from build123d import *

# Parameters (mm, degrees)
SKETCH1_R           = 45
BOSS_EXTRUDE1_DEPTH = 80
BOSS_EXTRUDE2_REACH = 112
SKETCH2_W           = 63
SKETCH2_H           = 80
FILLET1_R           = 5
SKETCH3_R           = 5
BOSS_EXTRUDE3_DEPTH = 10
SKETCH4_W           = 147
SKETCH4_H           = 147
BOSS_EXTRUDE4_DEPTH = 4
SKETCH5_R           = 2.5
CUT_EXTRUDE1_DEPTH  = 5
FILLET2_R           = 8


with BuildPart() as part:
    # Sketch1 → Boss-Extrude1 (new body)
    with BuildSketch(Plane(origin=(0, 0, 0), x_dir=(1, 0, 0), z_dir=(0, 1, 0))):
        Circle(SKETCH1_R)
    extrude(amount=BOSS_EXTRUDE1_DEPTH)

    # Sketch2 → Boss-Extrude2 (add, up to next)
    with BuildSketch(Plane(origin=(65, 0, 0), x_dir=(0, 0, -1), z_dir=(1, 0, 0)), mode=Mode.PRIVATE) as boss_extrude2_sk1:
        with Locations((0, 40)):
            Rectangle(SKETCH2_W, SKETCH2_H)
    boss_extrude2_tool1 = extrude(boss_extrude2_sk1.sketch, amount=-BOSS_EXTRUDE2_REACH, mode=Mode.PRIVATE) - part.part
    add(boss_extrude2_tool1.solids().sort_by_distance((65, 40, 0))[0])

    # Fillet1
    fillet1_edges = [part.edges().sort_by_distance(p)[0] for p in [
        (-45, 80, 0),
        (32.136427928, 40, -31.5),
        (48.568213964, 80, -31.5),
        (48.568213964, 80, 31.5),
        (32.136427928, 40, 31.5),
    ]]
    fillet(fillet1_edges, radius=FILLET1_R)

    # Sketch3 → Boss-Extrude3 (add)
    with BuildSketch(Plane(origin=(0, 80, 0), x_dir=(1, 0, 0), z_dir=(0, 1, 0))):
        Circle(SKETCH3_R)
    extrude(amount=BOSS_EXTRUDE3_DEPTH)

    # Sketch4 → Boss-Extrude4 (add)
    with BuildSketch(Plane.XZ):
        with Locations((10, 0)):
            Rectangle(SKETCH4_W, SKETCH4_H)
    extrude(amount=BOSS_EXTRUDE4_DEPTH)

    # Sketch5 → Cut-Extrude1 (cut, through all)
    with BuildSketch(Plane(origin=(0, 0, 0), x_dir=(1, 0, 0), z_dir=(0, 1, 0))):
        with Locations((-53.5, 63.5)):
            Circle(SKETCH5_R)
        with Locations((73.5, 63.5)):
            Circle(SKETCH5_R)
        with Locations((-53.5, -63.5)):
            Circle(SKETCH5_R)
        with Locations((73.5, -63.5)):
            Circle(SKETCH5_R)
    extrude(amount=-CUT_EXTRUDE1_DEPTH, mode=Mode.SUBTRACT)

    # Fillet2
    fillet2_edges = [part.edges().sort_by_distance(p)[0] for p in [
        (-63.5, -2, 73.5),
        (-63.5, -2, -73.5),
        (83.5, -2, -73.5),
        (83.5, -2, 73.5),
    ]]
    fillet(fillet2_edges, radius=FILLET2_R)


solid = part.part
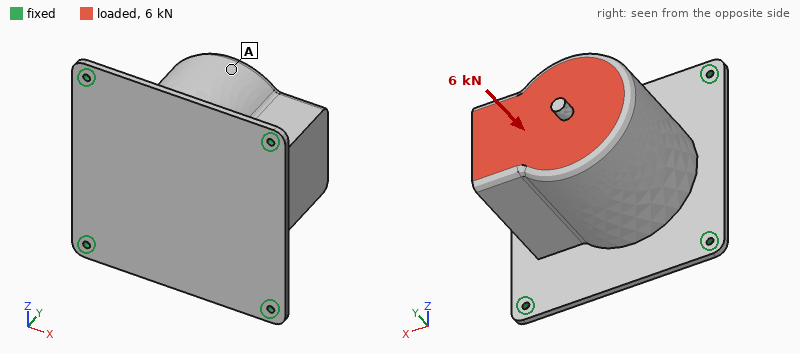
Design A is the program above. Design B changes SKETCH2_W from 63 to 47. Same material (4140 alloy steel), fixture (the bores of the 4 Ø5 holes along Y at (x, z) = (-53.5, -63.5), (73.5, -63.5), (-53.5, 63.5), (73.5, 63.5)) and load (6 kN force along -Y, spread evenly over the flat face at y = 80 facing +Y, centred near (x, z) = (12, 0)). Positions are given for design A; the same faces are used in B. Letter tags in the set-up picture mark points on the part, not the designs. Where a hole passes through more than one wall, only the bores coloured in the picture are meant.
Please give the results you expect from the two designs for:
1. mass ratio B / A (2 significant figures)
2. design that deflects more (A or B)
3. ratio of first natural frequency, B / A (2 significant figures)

0.95
B
0.91
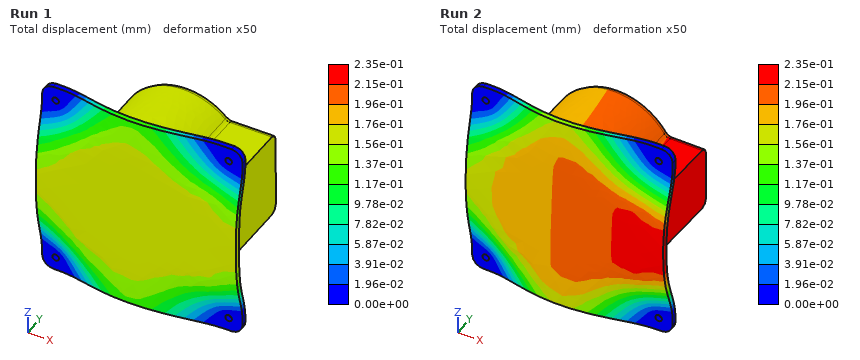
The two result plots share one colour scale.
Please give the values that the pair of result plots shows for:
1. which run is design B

Run 2
